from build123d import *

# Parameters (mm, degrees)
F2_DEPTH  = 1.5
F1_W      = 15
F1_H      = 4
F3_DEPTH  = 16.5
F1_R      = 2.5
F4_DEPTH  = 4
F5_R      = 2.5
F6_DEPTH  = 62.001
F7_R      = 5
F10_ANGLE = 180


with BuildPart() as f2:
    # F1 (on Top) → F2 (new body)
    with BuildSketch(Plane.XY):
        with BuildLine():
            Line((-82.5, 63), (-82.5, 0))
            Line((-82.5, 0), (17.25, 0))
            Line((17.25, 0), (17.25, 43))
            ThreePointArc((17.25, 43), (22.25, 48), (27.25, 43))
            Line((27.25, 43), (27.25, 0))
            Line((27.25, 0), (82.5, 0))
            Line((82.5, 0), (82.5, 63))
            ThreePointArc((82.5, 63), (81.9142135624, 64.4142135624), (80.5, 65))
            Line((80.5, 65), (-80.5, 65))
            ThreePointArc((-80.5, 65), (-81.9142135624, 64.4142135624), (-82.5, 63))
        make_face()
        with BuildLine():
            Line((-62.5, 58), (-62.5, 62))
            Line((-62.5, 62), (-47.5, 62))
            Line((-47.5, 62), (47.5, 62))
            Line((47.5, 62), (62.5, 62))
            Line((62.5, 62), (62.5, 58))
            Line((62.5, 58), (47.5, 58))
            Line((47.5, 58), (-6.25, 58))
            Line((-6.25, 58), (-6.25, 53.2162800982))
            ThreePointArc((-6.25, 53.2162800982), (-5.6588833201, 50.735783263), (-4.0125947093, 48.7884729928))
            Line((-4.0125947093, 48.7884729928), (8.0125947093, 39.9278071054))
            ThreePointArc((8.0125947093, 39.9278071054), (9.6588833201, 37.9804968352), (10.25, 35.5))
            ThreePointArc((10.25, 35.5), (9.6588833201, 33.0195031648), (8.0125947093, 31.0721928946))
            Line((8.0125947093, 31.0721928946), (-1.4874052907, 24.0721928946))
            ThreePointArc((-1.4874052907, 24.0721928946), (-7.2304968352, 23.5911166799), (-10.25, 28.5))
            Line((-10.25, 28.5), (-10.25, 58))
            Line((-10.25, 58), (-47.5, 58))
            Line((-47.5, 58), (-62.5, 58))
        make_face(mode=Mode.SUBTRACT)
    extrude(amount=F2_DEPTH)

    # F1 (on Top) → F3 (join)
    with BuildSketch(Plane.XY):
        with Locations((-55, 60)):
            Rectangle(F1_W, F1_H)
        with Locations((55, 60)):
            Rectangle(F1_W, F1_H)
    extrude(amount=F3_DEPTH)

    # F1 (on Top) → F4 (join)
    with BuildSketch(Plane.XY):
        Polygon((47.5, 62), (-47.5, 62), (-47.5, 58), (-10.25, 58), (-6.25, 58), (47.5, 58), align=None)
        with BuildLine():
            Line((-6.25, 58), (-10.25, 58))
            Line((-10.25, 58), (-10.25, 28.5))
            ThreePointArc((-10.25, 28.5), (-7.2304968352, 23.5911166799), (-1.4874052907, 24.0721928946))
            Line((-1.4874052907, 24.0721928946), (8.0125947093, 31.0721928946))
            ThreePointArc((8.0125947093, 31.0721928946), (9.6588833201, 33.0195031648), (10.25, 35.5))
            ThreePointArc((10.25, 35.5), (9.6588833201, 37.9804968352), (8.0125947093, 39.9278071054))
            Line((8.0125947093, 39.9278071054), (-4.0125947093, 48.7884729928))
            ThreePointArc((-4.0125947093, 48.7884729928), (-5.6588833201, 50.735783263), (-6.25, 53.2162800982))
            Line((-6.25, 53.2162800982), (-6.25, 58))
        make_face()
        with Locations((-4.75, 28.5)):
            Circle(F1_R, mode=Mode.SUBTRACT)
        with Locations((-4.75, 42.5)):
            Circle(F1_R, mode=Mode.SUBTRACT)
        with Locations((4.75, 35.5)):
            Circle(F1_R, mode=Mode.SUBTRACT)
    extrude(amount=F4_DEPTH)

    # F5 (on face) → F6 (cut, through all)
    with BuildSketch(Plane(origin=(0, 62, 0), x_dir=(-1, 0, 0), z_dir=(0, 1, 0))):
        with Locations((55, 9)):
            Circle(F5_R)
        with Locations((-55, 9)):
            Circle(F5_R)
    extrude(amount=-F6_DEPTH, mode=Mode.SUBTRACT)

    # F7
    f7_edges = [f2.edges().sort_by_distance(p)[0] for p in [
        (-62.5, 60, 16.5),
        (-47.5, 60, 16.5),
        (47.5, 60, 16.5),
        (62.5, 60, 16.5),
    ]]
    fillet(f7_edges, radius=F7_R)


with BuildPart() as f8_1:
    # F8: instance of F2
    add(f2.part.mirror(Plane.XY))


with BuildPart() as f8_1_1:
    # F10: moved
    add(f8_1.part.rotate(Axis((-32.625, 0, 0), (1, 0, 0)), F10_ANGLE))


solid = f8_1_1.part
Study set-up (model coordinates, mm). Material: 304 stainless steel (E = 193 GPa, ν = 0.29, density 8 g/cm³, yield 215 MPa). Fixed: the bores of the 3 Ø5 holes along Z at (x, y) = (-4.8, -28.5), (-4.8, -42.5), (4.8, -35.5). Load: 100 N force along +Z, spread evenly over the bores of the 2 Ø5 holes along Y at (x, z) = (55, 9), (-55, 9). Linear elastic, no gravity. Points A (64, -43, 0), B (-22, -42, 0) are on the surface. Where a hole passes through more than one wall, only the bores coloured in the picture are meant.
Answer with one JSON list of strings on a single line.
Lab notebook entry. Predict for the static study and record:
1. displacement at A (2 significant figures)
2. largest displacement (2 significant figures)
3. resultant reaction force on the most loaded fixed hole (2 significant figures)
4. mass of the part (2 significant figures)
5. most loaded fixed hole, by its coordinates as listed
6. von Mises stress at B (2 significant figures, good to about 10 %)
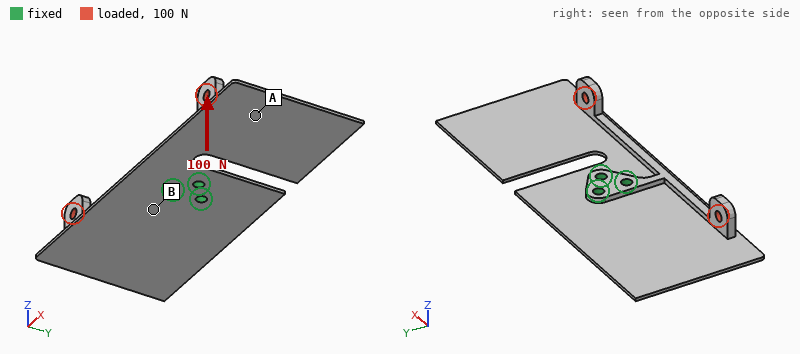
["0.53 mm", "0.83 mm", "77 N", "150 g", "(-4.8, -42.5)", "27 MPa"]
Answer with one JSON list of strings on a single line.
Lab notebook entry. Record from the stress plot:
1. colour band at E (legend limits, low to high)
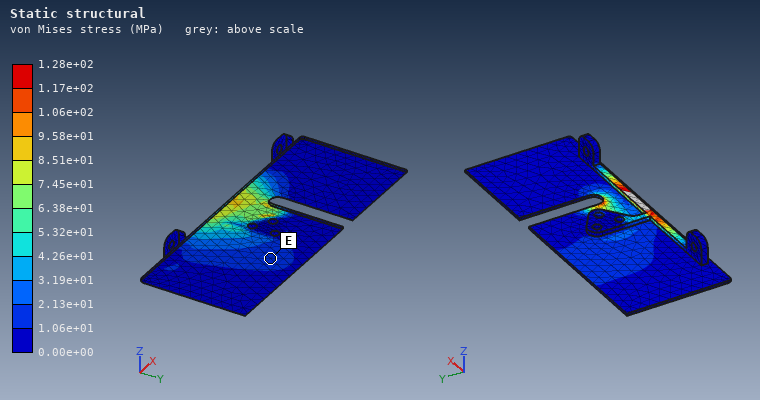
["1.06e+01 to 2.13e+01 MPa"]
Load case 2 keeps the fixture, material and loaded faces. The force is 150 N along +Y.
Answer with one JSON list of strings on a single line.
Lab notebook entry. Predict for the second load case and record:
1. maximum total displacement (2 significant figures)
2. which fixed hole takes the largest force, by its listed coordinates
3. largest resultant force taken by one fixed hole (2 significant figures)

["0.30 mm", "(4.8, -35.5)", "110 N"]
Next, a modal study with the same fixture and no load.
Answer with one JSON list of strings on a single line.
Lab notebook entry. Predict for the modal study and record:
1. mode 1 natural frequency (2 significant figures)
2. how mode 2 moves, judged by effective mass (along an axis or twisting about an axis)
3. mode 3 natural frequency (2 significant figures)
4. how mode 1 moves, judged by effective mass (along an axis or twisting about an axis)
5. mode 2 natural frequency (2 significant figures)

["170 Hz", "along Z", "340 Hz", "along Z", "280 Hz"]
